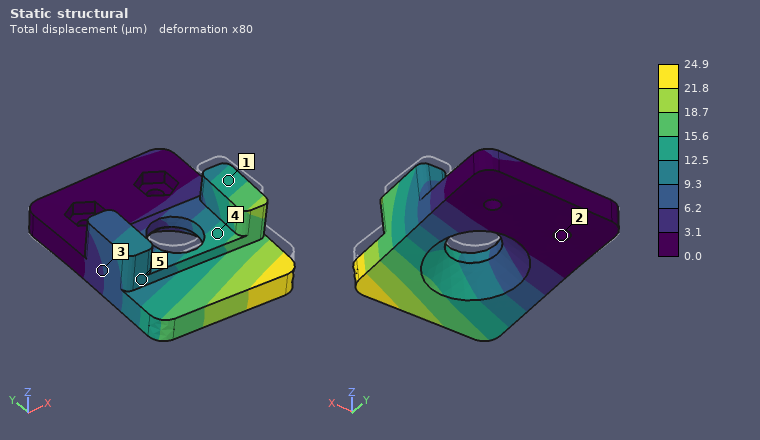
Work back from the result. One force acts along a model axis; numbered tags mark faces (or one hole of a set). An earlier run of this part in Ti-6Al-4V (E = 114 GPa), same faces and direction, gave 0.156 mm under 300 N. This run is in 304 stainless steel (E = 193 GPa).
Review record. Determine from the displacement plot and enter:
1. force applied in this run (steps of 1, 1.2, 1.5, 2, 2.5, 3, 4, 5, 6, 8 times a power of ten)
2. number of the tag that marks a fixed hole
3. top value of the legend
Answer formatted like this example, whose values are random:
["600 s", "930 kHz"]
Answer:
["80 N", "2", "24.9 µm"]
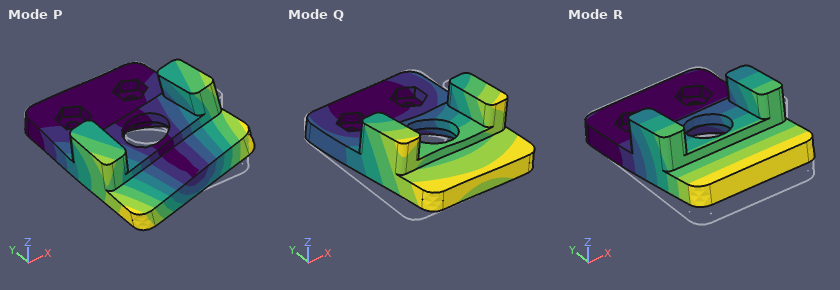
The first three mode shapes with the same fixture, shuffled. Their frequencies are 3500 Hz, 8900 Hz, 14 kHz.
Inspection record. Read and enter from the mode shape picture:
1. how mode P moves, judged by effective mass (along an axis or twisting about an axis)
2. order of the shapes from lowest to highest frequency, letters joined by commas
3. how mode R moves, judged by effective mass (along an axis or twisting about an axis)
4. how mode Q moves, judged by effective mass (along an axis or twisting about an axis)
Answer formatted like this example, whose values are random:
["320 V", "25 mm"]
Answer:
["twisting about Y", "R, P, Q", "along Z", "along X"]
